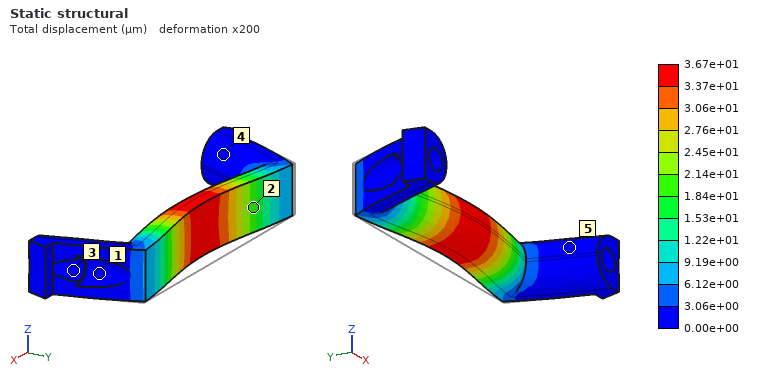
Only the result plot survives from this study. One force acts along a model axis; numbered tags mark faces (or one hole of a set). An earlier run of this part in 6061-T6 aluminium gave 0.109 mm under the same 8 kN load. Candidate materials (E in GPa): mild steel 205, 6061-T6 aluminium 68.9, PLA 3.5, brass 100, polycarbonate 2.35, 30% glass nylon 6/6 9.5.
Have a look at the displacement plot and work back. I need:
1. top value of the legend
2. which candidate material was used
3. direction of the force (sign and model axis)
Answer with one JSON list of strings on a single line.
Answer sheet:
["3.67e+01 µm", "mild steel", "-Y"]
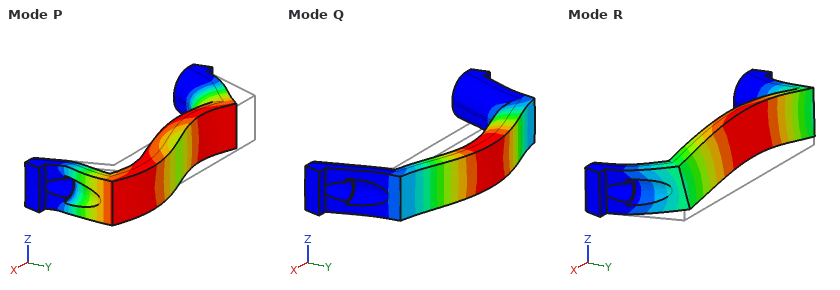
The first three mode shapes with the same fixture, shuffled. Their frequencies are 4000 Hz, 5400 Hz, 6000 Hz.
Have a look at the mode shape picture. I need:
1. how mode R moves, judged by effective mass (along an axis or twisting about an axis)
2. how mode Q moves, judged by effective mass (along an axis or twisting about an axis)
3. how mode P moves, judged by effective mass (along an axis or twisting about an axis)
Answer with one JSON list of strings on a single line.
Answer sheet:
["along Z", "along Y", "along X"]
